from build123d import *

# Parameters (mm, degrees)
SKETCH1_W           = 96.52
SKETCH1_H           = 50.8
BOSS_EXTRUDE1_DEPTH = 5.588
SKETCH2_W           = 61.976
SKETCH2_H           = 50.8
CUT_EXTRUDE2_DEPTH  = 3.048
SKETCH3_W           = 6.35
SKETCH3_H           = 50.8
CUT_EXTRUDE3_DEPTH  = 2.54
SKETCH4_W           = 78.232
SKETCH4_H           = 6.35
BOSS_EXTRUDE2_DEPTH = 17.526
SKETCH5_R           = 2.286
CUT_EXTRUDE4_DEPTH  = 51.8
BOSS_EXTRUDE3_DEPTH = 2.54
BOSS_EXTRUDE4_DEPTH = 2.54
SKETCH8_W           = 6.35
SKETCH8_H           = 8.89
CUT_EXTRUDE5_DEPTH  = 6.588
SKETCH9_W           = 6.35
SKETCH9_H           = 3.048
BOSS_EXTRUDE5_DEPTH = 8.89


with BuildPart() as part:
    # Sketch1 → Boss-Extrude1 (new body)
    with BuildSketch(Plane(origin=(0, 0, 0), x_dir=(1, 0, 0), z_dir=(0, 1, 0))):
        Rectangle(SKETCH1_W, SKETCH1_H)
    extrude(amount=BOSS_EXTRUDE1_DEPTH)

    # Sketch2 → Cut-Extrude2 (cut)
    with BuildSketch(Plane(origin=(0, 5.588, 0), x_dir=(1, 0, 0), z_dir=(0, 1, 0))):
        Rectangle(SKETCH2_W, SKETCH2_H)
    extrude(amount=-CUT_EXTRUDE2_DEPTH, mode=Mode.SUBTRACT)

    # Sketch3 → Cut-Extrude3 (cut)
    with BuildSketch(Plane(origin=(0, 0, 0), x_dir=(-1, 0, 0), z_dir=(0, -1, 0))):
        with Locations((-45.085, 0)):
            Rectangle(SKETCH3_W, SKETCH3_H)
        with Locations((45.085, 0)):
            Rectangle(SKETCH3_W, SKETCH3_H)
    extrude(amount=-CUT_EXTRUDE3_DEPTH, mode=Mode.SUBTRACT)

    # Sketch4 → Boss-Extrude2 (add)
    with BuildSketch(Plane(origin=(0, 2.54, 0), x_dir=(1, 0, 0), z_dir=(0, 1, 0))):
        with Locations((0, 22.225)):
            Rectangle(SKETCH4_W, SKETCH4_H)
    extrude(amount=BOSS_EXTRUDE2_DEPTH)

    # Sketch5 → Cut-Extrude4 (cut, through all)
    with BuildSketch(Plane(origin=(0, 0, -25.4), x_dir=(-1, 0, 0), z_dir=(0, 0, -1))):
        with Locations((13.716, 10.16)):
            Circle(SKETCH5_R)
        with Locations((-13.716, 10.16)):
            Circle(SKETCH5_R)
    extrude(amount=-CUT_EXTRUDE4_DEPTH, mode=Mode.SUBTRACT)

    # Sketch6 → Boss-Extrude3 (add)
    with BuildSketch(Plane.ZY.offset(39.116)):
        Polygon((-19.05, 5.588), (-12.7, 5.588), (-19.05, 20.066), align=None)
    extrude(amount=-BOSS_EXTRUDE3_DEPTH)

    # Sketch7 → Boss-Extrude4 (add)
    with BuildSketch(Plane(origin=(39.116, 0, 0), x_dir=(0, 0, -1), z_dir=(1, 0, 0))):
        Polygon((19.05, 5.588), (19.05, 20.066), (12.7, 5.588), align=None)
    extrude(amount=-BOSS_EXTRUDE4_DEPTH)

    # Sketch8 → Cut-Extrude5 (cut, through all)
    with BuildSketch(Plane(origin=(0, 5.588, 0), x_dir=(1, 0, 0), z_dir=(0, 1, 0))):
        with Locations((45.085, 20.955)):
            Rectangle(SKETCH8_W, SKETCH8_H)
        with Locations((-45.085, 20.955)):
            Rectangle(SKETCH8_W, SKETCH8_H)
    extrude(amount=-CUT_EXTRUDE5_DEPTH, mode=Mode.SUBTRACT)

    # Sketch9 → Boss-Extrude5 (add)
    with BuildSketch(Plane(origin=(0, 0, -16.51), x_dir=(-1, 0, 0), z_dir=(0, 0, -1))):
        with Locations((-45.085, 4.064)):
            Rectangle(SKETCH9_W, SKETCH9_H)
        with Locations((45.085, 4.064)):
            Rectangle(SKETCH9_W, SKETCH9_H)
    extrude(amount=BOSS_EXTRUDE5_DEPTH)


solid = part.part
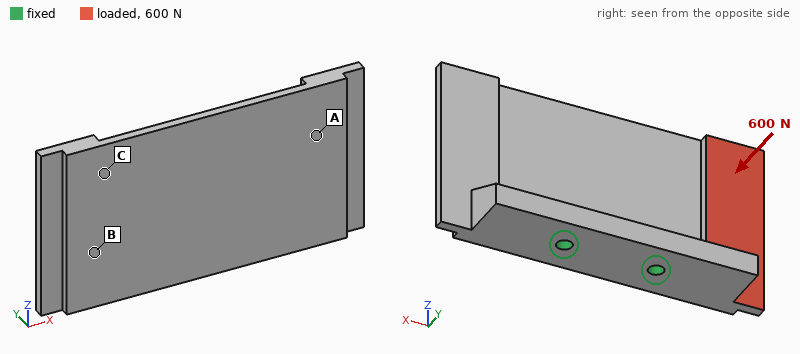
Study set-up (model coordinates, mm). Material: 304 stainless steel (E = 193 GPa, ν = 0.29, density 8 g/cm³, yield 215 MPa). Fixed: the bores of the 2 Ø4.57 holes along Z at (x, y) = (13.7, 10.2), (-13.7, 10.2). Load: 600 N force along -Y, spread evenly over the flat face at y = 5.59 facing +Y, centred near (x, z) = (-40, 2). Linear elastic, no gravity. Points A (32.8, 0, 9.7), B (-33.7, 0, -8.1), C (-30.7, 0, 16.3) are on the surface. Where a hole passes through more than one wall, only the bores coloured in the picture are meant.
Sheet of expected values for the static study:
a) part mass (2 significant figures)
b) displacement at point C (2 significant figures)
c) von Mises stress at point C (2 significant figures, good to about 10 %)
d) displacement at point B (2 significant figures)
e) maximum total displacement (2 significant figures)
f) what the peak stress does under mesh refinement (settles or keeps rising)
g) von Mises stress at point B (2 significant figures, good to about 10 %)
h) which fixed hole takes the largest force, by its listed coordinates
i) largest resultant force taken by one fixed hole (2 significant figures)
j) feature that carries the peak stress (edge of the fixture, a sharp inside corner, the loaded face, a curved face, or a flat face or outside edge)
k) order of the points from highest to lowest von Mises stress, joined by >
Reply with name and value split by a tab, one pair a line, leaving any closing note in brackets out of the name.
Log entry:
part mass	200 g
displacement at point C	0.15 mm
von Mises stress at point C	34 MPa
displacement at point B	0.047 mm
maximum total displacement	0.23 mm
what the peak stress does under mesh refinement	keeps rising
von Mises stress at point B	60 MPa
which fixed hole takes the largest force, by its listed coordinates	(-13.7, 10.2)
largest resultant force taken by one fixed hole	1.0 kN
feature that carries the peak stress	edge of the fixture
order of the points from highest to lowest von Mises stress, joined by >	B > C > A
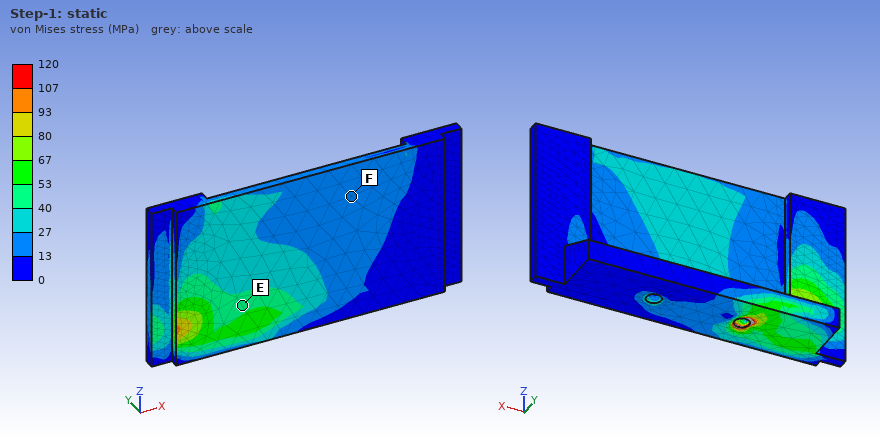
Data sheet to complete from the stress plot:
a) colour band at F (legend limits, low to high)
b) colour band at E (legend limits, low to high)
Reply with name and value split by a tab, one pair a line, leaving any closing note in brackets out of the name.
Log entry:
colour band at F	13 to 27 MPa
colour band at E	40 to 53 MPa
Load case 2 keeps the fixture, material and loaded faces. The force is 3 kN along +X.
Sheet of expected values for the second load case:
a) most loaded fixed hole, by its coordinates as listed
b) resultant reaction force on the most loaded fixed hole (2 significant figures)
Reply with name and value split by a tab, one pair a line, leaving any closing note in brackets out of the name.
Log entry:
most loaded fixed hole, by its coordinates as listed	(-13.7, 10.2)
resultant reaction force on the most loaded fixed hole	2.8 kN
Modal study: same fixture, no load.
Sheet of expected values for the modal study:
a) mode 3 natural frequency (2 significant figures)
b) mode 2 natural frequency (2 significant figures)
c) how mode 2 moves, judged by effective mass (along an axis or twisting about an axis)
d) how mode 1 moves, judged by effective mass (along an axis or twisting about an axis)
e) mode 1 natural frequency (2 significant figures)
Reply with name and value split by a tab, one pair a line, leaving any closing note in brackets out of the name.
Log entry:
mode 3 natural frequency	3300 Hz
mode 2 natural frequency	1700 Hz
how mode 2 moves, judged by effective mass	twisting about Z
how mode 1 moves, judged by effective mass	along Y
mode 1 natural frequency	1300 Hz
